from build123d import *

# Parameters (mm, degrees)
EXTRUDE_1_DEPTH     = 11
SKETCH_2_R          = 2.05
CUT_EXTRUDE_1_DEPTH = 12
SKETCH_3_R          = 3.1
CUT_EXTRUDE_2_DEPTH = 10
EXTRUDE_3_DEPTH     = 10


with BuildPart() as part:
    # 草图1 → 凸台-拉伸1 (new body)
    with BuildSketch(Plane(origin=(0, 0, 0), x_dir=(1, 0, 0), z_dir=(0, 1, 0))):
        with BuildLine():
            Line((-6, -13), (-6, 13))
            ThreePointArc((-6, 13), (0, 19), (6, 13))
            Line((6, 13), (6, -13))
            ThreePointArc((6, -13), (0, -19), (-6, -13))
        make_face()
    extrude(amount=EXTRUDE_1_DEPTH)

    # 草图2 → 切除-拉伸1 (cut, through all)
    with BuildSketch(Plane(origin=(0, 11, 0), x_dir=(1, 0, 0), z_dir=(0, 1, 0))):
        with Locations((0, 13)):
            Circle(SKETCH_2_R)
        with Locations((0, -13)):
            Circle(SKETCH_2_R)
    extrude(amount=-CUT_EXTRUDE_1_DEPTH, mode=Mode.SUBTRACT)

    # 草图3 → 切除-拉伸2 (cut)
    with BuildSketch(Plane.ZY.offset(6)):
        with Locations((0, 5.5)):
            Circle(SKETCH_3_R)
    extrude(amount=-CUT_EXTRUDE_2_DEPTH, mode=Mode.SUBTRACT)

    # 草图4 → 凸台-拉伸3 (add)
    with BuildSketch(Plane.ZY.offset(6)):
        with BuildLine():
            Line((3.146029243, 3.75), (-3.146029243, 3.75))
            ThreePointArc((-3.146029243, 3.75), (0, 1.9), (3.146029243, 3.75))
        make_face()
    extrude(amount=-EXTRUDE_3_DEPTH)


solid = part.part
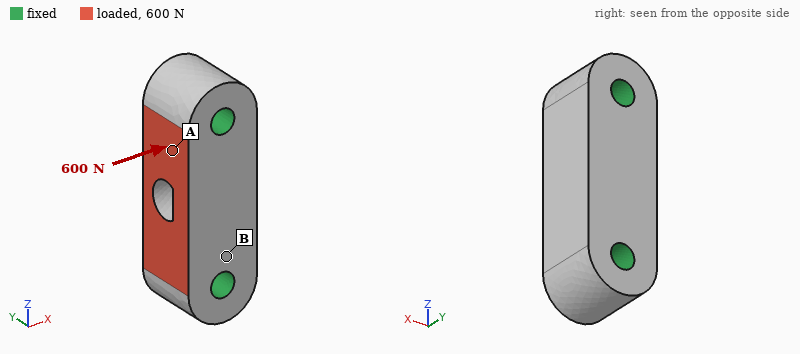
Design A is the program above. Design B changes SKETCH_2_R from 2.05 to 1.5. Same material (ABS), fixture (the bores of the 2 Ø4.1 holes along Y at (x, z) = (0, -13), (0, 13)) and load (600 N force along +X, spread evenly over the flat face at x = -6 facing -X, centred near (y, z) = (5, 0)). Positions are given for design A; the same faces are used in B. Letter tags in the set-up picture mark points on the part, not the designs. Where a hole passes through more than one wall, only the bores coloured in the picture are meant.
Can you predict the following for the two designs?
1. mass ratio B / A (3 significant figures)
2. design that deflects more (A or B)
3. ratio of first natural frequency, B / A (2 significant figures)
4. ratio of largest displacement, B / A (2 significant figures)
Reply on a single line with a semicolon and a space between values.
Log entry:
1.03; B; 0.87; 1.2
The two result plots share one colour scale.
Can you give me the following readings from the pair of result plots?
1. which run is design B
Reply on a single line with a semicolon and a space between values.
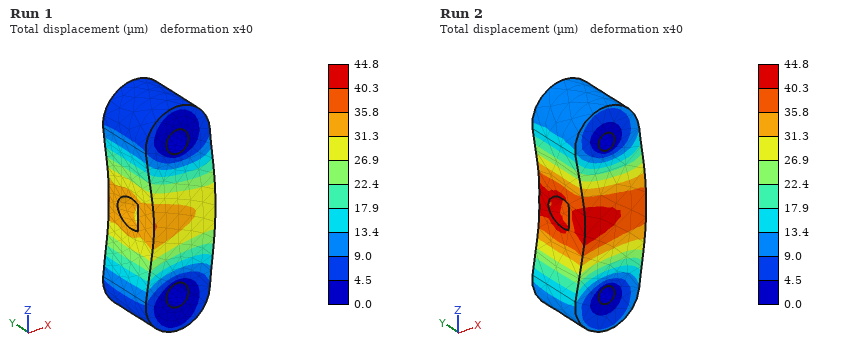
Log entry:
Run 2
